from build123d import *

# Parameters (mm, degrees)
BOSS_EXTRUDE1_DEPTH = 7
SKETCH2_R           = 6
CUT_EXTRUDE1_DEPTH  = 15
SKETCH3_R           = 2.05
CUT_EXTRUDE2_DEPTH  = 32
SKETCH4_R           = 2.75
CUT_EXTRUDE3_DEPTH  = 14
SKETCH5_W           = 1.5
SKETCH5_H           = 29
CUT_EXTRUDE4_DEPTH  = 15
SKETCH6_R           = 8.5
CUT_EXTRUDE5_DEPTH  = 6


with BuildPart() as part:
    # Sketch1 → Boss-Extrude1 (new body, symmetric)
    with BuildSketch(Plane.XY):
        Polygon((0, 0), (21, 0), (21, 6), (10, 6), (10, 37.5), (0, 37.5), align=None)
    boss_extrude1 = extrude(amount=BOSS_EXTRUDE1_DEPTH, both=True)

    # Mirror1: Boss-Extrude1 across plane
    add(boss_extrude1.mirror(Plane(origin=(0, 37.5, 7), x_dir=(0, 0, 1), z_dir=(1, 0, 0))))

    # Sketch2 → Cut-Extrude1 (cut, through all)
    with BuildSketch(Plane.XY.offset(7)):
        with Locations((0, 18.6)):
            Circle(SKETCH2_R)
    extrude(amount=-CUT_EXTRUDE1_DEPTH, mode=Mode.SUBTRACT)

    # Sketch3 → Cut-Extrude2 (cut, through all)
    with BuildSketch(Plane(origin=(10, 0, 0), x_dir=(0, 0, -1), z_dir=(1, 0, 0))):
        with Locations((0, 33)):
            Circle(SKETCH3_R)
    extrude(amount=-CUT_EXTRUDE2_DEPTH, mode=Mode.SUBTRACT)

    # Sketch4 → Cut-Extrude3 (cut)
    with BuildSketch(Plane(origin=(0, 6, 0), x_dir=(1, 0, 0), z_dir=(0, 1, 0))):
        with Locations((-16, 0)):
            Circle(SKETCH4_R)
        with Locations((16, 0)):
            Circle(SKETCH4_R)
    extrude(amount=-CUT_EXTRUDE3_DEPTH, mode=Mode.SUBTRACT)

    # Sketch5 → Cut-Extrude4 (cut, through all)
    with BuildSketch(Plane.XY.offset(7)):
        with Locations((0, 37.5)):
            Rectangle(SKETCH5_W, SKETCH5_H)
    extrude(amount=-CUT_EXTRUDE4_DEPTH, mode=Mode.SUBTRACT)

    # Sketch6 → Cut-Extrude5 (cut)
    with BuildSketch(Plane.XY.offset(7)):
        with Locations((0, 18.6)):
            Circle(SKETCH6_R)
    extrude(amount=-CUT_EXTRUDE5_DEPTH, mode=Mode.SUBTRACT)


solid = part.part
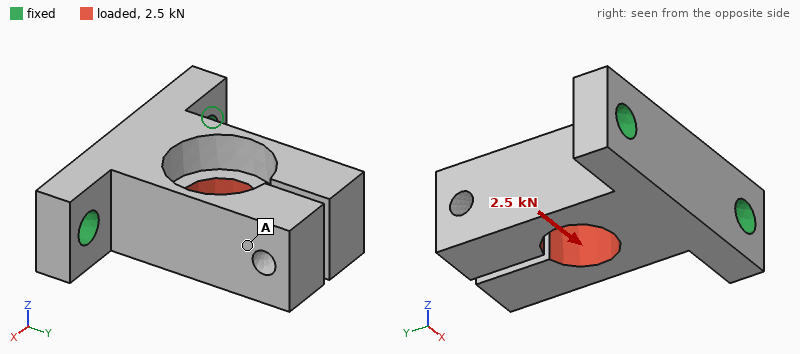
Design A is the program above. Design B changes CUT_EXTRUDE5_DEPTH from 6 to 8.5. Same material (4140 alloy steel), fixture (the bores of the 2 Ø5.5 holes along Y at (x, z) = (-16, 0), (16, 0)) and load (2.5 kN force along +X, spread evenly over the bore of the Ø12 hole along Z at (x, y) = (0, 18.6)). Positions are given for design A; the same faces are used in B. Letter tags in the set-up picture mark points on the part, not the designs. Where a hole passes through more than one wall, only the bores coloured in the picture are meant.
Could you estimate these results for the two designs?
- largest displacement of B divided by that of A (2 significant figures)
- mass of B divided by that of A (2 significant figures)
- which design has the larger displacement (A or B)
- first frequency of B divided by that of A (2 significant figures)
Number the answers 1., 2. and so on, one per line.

1. 1.3
2. 0.97
3. B
4. 0.86
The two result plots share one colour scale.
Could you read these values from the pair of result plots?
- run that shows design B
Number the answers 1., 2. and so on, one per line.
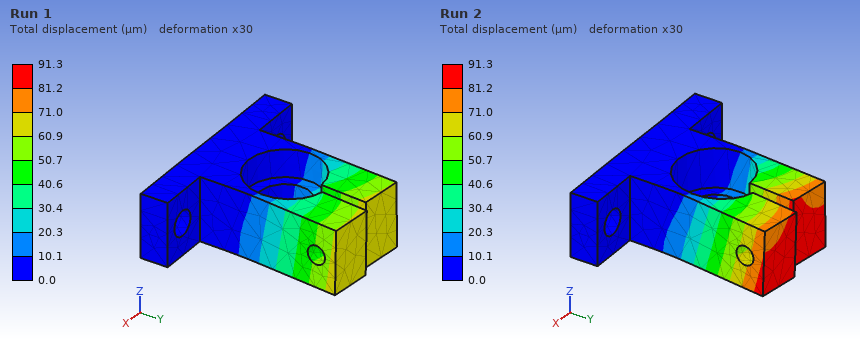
1. Run 2
